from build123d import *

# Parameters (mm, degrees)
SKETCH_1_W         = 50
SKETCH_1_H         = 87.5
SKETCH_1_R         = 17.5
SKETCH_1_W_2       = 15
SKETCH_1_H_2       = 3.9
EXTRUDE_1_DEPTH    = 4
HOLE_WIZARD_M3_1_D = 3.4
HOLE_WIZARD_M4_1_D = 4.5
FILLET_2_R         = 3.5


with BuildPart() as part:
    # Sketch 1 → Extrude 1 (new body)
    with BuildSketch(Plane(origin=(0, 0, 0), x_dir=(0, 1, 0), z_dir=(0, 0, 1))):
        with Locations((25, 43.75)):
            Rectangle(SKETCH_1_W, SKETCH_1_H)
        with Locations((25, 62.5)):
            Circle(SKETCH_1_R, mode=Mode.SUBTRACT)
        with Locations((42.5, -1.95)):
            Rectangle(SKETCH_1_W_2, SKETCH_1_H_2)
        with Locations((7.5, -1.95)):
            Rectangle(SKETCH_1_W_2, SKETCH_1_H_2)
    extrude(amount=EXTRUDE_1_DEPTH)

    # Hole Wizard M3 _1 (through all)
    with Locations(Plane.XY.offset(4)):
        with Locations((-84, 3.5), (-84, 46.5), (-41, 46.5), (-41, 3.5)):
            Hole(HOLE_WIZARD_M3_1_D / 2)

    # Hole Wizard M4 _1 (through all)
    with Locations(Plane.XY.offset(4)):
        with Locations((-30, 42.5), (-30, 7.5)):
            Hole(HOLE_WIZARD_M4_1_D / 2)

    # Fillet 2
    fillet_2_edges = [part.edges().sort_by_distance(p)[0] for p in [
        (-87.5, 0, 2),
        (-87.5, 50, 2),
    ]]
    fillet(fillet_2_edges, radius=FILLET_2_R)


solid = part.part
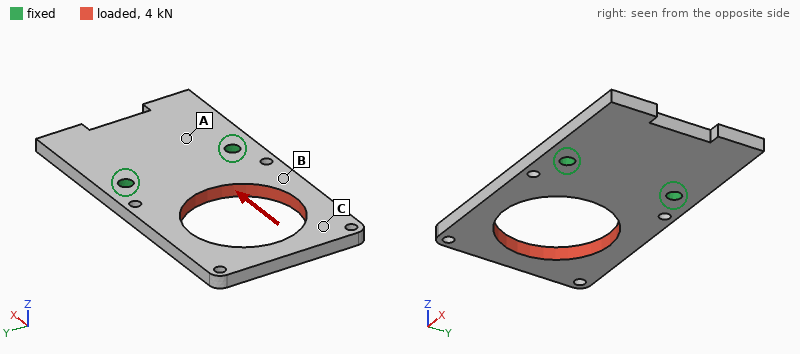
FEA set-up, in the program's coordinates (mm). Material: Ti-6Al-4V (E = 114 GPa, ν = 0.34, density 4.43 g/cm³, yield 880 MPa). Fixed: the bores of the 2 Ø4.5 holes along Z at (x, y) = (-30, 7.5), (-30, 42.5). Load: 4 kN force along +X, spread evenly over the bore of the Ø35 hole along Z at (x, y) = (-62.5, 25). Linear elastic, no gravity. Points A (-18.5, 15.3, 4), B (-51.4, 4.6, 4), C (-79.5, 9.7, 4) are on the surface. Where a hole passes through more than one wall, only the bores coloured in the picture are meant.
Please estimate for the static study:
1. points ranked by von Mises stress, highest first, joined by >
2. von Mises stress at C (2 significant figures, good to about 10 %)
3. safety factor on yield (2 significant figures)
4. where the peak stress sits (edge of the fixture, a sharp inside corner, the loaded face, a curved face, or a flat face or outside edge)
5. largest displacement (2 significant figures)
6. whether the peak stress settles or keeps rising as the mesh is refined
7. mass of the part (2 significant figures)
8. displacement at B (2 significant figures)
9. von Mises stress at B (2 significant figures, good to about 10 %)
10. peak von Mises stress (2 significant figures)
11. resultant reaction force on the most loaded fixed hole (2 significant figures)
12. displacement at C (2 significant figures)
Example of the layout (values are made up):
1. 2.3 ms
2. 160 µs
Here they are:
1. B > C > A
2. 18 MPa
3. 5.6
4. a curved face
5. 37 µm
6. settles
7. 61 g
8. 11 µm
9. 41 MPa
10. 160 MPa
11. 2.0 kN
12. 22 µm
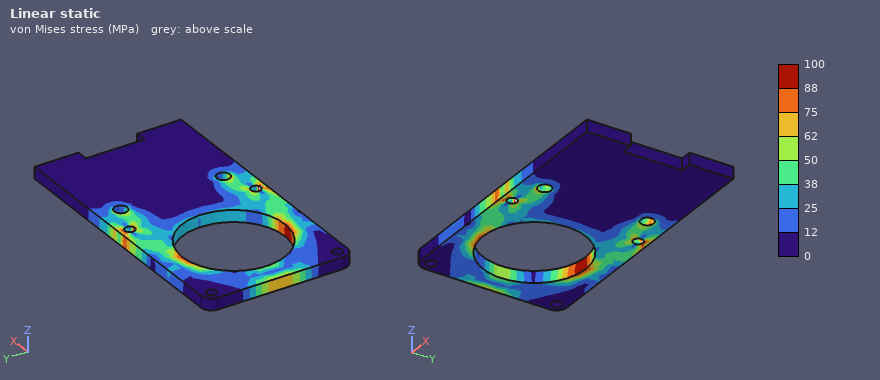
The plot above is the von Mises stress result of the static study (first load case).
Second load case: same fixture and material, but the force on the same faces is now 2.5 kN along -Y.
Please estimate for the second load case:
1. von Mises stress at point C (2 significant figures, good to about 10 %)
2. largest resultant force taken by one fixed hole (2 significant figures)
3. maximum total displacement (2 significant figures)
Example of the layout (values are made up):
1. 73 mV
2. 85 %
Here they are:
1. 14 MPa
2. 2.5 kN
3. 0.12 mm
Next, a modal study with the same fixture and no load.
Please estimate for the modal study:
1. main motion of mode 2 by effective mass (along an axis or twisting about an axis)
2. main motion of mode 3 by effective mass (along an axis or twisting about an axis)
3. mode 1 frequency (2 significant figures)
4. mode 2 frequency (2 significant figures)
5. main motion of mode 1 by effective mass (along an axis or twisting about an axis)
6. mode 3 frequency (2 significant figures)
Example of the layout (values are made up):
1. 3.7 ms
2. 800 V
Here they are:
1. twisting about X
2. along Z
3. 920 Hz
4. 2200 Hz
5. along Z
6. 3000 Hz
